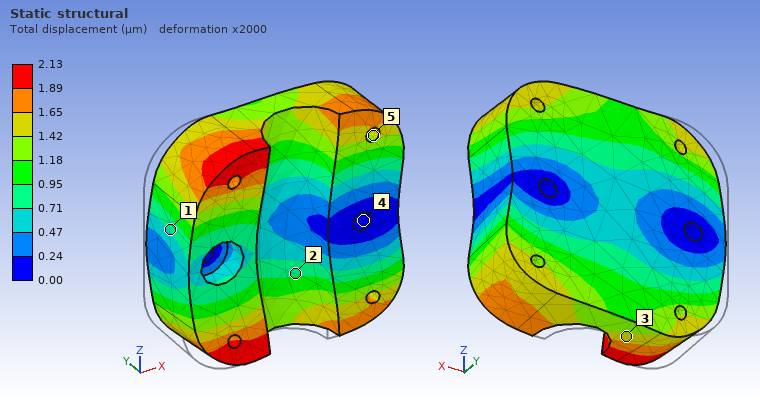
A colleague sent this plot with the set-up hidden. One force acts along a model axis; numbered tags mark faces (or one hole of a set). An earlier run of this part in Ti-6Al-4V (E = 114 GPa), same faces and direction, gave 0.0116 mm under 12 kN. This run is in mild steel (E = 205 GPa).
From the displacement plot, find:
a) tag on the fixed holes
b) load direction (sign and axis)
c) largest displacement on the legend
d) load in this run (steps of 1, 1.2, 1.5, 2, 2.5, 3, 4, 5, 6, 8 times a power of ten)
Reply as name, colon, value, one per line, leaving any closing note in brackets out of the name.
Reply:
tag on the fixed holes: 4
load direction: +X
largest displacement on the legend: 2.13 µm
load in this run: 4 kN
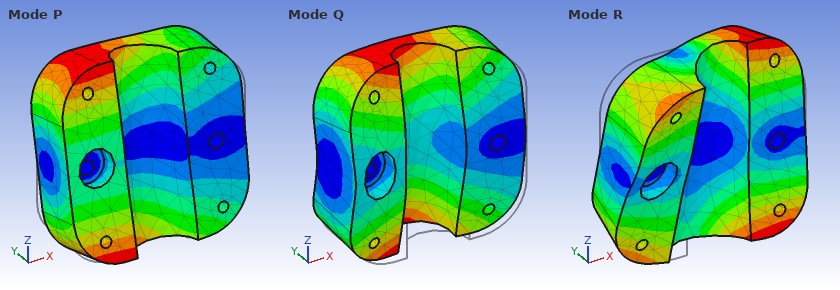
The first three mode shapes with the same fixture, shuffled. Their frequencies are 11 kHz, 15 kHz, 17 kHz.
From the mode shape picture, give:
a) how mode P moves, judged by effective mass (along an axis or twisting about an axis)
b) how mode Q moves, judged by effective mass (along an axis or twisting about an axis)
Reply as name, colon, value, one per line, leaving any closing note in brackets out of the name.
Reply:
how mode P moves, judged by effective mass: twisting about X
how mode Q moves, judged by effective mass: along Y
